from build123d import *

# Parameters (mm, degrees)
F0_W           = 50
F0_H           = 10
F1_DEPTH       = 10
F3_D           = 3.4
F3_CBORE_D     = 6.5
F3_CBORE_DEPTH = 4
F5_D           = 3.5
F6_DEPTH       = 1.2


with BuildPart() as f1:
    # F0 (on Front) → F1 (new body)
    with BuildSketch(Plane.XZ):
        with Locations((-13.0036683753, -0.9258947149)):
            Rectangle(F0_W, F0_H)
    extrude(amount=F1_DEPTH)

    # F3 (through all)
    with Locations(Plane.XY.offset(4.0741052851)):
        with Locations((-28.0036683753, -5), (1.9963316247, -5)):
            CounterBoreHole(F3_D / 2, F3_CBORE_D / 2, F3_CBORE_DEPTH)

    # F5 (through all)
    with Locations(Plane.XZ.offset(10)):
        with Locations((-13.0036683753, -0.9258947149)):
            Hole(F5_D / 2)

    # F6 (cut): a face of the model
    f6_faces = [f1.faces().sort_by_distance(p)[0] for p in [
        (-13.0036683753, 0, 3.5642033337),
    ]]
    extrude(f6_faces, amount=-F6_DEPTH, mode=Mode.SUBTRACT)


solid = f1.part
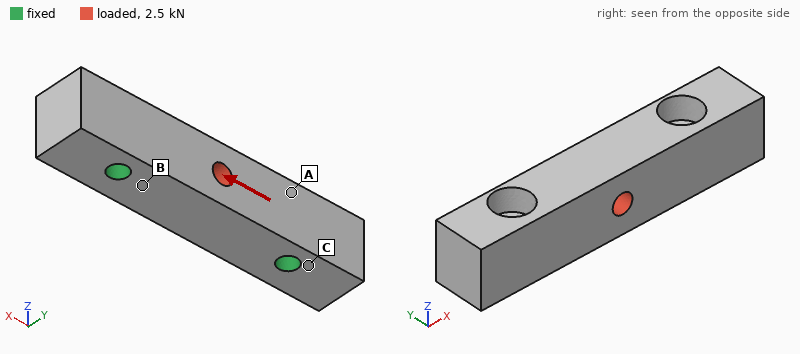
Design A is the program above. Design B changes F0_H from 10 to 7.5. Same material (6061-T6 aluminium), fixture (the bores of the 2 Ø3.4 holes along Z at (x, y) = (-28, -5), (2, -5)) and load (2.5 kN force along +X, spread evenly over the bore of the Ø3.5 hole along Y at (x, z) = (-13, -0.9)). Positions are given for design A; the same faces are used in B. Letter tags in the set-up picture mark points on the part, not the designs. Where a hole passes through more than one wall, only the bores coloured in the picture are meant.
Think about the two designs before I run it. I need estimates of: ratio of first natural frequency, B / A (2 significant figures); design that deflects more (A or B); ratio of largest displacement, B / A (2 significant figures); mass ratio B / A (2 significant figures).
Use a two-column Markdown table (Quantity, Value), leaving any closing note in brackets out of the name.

| Quantity | Value |
|---|---|
| ratio of first natural frequency, B / A | 1.1 |
| design that deflects more | B |
| ratio of largest displacement, B / A | 1.2 |
| mass ratio B / A | 0.73 |
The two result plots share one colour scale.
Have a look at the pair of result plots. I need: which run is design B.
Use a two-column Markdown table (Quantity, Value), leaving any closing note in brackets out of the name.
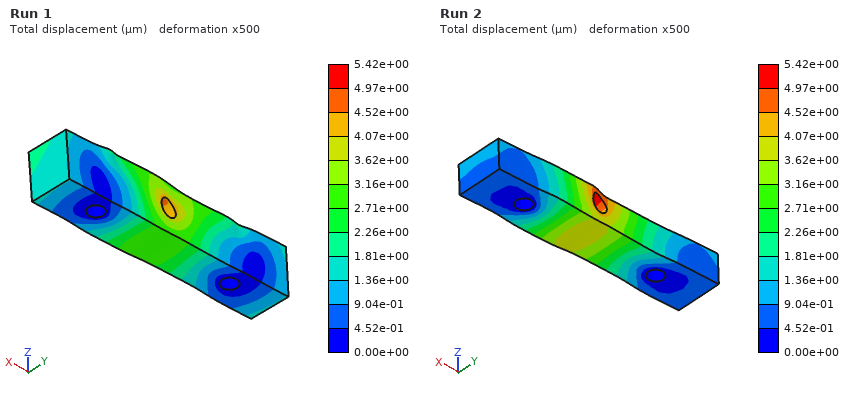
| Quantity | Value |
|---|---|
| which run is design B | Run 2 |
